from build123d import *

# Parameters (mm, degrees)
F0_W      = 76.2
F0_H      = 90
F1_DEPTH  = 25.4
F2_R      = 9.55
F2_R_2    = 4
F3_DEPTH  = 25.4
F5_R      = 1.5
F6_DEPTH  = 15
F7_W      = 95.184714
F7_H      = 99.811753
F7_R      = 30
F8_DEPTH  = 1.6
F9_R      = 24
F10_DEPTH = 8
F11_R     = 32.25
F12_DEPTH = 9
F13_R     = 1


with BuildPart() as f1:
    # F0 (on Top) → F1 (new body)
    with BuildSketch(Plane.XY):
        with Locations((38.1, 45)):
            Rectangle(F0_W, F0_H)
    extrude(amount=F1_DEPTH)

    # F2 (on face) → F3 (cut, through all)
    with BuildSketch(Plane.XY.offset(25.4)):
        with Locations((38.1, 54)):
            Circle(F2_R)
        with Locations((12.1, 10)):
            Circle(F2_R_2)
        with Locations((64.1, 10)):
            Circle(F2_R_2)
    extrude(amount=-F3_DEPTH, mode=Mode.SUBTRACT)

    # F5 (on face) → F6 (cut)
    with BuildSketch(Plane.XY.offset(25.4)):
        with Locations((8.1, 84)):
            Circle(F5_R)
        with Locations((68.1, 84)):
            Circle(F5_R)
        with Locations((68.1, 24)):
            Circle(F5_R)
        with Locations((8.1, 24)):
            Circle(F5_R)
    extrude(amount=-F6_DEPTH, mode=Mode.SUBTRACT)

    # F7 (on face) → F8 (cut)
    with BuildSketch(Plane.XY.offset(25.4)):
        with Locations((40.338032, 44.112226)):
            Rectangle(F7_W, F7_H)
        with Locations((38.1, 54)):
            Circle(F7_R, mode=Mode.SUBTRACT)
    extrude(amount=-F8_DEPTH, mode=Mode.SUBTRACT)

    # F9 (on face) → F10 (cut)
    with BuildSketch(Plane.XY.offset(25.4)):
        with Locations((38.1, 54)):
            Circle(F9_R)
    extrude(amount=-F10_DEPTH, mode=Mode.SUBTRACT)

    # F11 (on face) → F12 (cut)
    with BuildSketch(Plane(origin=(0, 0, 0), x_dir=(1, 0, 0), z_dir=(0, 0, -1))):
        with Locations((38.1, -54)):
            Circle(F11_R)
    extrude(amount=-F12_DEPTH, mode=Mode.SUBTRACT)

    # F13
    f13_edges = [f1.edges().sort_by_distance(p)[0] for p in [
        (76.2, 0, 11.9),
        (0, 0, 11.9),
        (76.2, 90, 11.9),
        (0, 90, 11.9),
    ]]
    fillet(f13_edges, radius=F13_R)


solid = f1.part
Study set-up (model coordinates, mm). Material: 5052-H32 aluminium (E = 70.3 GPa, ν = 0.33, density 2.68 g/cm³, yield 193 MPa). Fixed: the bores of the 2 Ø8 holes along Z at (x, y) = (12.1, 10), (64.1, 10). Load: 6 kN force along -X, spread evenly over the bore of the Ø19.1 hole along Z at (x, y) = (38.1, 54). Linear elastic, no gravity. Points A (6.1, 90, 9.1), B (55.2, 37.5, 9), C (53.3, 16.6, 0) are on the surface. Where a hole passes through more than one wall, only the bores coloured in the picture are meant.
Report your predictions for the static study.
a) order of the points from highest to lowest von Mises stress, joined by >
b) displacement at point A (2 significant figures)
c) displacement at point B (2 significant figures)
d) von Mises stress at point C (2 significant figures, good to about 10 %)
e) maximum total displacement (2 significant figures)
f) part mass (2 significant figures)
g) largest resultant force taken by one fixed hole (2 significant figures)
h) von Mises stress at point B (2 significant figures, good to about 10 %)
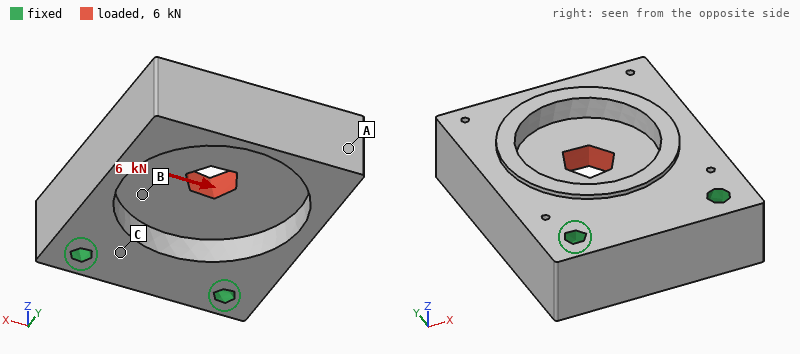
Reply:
B > C > A
28 µm
8.8 µm
7.9 MPa
29 µm
320 g
5.4 kN
16 MPa
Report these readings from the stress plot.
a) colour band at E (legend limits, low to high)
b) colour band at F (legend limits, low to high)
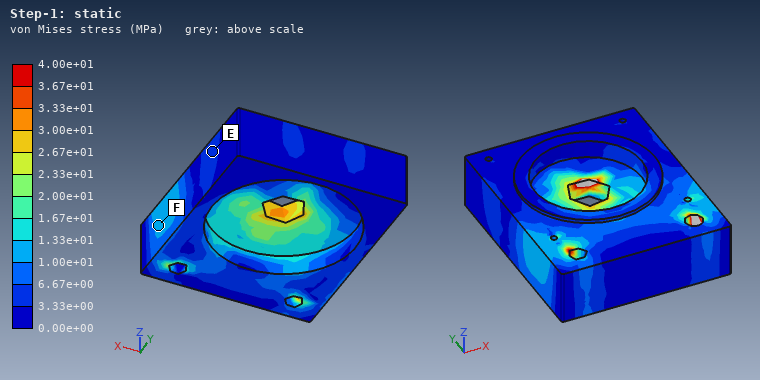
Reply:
3.33e+00 to 6.67e+00 MPa
1.00e+01 to 1.33e+01 MPa
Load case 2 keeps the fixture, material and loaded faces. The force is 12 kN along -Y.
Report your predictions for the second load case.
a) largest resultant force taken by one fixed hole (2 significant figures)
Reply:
6.1 kN
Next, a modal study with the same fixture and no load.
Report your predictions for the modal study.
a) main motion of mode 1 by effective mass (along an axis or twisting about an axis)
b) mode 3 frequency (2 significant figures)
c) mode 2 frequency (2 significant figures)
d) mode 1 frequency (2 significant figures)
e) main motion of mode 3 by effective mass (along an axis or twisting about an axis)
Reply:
along Z
5500 Hz
4300 Hz
2300 Hz
along X
